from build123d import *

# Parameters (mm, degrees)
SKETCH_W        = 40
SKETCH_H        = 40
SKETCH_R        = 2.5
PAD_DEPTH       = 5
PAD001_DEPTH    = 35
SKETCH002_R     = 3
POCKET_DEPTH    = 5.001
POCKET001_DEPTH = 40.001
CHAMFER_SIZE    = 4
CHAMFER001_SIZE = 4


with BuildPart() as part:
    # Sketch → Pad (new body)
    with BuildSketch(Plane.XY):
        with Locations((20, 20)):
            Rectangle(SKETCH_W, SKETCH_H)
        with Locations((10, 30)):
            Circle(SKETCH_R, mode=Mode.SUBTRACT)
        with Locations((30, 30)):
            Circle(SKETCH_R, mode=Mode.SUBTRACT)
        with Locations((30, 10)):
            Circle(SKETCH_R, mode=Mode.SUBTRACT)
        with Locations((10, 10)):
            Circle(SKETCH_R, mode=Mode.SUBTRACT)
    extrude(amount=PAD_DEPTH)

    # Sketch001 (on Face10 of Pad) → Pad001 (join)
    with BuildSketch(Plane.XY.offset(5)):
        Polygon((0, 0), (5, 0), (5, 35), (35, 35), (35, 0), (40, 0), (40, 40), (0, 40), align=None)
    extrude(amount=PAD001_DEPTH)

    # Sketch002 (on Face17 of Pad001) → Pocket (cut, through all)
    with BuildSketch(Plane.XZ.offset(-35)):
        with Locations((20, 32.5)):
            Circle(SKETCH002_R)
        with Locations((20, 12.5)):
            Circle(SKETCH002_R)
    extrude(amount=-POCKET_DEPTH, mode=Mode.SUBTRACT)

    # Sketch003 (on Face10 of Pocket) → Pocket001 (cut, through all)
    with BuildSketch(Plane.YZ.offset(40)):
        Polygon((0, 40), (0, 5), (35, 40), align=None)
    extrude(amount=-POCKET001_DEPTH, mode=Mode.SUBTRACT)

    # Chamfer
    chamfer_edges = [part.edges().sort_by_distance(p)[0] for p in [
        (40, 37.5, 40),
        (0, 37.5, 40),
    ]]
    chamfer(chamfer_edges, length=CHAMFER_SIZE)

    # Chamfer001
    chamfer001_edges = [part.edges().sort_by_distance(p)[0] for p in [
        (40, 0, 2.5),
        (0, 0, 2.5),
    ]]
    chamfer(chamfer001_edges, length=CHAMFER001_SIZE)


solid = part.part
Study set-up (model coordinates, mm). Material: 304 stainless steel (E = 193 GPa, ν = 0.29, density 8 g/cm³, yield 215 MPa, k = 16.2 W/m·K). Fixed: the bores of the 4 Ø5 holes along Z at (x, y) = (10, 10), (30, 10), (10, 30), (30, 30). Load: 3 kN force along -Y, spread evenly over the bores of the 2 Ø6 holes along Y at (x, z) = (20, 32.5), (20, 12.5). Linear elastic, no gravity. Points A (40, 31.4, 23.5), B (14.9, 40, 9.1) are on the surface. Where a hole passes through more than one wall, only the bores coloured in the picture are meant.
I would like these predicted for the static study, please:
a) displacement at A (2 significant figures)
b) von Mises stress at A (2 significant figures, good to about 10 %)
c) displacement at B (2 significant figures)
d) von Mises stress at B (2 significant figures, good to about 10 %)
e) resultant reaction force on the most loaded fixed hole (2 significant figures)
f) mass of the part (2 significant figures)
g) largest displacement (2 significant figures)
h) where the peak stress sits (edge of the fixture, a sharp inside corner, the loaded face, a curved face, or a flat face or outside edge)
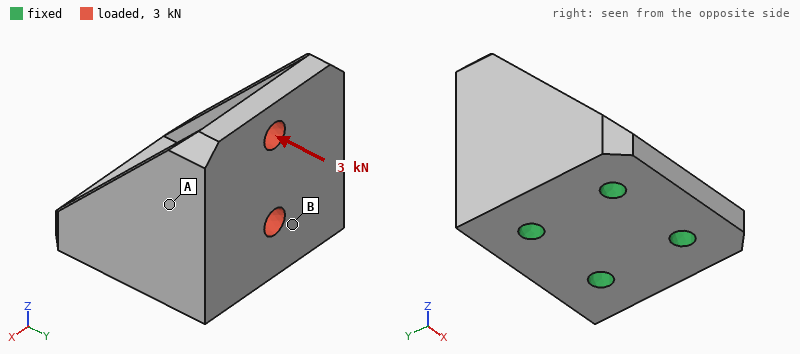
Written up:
9.5 µm
27 MPa
11 µm
57 MPa
1.5 kN
160 g
48 µm
the loaded face
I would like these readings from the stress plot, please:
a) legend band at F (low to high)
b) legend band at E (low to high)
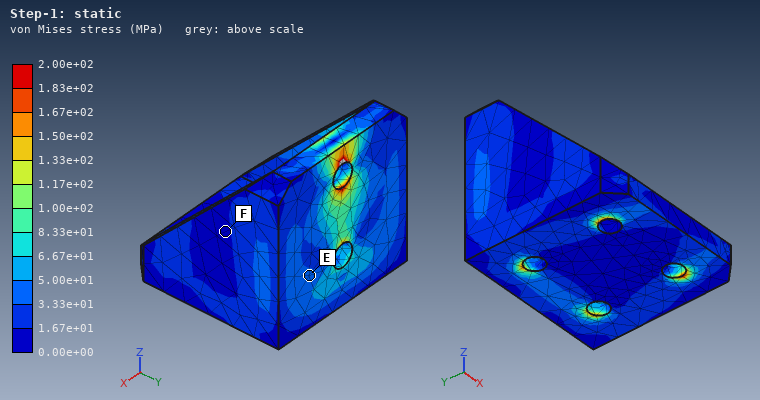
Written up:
0.00e+00 to 1.67e+01 MPa
3.33e+01 to 5.00e+01 MPa
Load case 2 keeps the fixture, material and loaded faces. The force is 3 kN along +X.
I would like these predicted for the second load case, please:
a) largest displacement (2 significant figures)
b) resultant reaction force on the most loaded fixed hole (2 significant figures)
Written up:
26 µm
2.8 kN
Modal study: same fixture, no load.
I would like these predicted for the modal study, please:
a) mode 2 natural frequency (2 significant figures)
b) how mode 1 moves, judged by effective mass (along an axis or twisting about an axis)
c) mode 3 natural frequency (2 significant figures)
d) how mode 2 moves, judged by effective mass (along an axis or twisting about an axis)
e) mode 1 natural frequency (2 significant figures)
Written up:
7500 Hz
along X
13 kHz
along Y
6700 Hz
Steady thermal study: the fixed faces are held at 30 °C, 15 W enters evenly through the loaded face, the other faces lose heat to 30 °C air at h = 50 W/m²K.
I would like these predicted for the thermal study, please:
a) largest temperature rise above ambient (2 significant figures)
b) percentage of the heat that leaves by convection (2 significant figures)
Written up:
64 K
48 %
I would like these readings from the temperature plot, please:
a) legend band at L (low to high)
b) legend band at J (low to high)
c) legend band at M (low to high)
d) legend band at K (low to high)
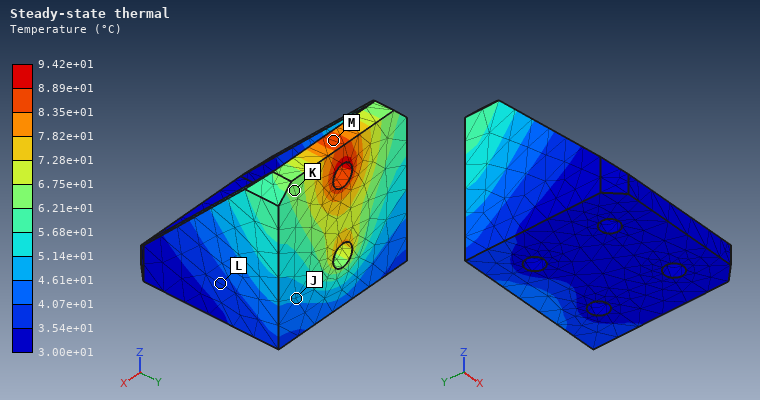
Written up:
3.54e+01 to 4.07e+01 °C
4.61e+01 to 5.14e+01 °C
8.35e+01 to 8.89e+01 °C
6.21e+01 to 6.75e+01 °C
